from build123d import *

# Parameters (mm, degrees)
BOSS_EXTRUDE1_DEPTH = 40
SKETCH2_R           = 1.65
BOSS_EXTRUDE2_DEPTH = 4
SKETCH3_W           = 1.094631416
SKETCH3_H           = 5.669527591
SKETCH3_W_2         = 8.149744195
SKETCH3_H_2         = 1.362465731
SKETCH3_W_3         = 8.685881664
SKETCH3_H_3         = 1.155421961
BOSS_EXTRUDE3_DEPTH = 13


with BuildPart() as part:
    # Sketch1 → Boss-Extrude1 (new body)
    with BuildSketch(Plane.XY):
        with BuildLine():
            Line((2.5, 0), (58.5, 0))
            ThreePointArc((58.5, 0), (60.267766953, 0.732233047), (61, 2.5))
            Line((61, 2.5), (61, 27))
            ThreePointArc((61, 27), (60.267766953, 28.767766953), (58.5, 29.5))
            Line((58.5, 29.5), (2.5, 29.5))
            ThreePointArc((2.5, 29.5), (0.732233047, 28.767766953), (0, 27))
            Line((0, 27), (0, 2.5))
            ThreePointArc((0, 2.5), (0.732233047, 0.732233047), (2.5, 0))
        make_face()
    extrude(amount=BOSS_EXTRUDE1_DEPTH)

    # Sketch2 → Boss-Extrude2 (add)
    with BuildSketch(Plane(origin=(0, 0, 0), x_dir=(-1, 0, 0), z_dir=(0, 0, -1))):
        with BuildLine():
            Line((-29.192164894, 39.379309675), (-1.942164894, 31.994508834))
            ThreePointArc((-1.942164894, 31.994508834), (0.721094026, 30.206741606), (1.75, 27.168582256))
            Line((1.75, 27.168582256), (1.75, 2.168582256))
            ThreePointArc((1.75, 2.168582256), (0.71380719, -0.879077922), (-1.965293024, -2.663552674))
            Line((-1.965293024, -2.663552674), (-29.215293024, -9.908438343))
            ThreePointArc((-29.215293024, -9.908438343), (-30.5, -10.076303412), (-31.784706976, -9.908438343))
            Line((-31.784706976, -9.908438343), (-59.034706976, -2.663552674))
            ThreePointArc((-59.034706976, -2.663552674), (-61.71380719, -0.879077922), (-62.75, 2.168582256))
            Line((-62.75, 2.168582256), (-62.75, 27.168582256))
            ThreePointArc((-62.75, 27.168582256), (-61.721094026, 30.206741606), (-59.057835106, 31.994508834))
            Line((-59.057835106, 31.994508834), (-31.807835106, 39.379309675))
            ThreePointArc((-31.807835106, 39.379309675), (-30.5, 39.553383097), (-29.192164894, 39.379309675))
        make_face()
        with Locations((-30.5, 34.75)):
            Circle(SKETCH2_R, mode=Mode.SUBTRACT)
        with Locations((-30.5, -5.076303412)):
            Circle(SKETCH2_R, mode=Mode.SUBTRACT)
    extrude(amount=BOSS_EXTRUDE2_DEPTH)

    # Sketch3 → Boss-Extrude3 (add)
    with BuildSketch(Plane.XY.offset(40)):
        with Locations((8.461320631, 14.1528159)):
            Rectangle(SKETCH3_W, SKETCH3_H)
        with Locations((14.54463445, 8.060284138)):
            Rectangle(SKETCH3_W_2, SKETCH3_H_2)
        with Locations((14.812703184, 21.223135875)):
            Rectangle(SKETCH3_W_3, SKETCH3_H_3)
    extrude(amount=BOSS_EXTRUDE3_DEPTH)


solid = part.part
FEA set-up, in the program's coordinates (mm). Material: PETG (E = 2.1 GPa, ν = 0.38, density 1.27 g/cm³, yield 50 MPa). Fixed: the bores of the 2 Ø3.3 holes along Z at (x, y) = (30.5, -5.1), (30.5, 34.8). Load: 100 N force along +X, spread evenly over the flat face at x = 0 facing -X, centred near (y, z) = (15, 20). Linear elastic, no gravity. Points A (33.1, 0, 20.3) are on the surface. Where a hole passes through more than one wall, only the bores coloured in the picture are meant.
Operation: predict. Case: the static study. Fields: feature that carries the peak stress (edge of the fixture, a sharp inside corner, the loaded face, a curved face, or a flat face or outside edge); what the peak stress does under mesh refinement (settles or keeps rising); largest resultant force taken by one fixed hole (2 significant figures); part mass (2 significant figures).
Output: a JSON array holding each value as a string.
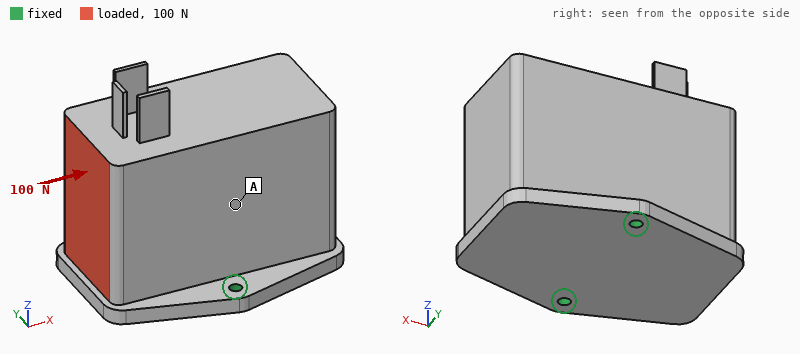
["edge of the fixture", "keeps rising", "50 N", "100 g"]
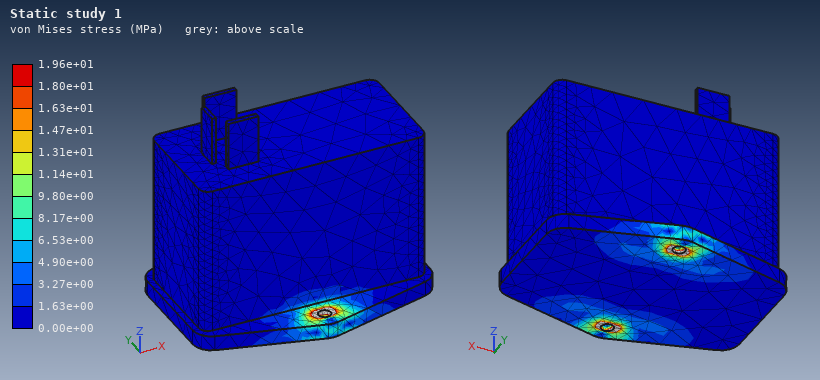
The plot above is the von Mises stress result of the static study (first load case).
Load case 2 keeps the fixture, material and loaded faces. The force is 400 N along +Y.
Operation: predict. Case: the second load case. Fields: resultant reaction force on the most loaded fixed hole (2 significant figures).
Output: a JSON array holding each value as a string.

["440 N"]
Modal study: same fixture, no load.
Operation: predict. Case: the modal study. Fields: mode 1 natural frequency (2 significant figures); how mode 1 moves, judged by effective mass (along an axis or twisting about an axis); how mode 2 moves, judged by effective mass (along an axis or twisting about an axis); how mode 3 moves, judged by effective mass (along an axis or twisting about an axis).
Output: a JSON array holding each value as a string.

["180 Hz", "along X", "along Y", "along Z"]
